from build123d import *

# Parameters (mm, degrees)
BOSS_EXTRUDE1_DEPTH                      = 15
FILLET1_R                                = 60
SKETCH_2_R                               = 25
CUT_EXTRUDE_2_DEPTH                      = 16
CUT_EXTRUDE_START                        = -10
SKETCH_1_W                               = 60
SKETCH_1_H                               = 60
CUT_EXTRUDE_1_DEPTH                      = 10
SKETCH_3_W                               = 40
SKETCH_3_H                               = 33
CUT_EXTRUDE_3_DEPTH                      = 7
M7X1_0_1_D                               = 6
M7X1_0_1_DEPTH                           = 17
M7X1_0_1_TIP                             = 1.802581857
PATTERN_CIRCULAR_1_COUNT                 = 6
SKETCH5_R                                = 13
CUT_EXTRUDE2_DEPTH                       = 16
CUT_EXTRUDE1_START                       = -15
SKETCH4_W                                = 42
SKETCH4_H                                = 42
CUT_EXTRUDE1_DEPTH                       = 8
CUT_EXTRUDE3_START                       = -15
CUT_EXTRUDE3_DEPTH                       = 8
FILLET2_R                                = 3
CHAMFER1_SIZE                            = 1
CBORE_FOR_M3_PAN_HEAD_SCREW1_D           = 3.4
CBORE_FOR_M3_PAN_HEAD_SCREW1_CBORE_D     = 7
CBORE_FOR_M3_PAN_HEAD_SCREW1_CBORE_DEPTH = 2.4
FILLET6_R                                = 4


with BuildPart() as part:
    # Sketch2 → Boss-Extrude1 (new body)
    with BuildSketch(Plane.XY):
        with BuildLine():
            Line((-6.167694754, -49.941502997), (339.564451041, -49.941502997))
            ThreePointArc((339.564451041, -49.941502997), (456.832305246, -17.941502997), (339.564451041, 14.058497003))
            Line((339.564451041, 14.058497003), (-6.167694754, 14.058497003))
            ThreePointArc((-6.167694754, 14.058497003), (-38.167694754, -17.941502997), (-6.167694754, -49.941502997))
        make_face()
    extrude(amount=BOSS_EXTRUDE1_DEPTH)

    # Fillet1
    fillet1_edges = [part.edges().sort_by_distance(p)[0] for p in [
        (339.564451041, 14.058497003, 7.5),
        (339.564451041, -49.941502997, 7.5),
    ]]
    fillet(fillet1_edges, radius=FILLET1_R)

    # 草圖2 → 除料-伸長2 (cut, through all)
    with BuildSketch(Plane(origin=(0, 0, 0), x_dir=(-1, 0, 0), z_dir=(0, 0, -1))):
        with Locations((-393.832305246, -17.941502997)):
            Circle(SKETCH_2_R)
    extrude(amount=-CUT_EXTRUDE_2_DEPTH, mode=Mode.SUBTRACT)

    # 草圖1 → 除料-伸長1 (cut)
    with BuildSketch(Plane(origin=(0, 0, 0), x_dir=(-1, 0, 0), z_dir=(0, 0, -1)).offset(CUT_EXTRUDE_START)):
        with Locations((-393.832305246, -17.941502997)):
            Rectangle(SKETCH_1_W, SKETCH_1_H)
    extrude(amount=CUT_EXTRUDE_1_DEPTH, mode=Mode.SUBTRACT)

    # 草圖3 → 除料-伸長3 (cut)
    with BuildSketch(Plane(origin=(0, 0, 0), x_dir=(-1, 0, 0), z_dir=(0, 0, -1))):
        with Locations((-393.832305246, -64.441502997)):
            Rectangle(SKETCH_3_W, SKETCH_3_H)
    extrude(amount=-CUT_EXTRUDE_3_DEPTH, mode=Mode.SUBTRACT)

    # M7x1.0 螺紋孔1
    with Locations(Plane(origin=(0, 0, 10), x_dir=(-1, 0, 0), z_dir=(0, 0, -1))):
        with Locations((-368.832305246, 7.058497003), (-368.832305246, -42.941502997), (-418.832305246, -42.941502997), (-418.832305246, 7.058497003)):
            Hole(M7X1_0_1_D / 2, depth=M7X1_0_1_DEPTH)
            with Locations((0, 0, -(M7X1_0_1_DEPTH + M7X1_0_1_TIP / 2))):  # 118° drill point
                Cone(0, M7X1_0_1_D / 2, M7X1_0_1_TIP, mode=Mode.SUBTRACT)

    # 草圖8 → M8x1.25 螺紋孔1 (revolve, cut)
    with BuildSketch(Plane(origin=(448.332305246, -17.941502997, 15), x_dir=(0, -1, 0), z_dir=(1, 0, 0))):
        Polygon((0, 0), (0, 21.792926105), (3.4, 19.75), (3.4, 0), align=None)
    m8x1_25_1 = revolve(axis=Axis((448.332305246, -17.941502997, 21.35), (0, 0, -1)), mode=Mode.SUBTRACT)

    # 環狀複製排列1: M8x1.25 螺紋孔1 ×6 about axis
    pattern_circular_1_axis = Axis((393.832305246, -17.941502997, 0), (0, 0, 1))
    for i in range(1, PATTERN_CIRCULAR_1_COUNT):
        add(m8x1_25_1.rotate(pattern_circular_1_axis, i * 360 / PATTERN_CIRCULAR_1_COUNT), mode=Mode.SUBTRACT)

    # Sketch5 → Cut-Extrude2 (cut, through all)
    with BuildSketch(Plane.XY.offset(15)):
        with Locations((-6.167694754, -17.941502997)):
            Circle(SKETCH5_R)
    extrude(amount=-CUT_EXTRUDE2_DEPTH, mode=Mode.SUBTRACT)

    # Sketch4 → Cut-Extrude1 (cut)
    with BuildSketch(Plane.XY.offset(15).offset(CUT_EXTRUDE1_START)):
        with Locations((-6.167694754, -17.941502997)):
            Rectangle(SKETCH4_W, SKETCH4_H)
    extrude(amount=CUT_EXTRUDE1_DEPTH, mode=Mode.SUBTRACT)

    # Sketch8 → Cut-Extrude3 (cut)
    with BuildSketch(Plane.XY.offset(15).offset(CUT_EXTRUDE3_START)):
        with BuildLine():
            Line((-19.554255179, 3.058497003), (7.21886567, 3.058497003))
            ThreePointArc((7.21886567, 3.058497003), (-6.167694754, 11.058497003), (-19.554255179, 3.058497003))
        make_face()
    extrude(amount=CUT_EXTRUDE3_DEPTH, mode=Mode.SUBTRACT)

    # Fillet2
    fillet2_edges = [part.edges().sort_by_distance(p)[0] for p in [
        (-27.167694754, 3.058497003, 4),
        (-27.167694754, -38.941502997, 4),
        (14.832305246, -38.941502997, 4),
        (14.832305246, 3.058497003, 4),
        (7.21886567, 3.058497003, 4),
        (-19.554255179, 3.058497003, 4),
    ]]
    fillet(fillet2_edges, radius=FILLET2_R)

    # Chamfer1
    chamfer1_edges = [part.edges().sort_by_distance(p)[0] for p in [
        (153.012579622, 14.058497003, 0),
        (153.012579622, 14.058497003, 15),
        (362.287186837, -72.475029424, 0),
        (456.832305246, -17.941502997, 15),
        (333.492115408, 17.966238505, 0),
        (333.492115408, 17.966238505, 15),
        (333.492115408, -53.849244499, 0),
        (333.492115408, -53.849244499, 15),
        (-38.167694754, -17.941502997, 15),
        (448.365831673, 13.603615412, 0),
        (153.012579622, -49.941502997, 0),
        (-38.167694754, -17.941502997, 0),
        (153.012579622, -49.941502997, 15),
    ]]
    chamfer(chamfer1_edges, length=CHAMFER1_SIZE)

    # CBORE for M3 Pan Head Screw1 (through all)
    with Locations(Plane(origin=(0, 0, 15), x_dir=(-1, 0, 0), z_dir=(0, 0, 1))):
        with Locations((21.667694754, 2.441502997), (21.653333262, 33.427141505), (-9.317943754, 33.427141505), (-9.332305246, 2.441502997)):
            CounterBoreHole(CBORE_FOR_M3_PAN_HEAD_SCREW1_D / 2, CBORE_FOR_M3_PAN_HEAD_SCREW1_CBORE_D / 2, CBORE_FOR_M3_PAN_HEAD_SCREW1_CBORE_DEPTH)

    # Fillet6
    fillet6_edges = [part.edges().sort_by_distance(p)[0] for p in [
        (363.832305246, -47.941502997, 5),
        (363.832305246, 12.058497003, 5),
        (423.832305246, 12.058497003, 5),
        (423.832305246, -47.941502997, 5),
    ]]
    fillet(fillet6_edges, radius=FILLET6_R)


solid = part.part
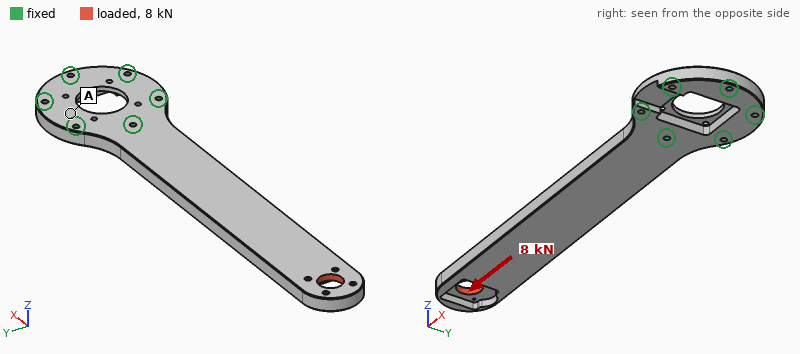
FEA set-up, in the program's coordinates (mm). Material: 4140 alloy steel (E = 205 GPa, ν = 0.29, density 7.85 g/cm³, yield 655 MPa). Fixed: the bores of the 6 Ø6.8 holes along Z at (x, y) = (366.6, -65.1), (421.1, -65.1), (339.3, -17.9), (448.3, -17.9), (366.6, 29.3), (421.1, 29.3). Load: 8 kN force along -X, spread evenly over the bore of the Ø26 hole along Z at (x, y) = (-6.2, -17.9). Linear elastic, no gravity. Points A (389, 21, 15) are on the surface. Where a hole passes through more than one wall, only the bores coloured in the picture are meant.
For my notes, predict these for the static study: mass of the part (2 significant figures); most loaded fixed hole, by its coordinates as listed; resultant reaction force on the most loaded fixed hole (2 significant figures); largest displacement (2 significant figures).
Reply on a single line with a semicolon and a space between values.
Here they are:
3.6 kg; (339.3, -17.9); 5.4 kN; 0.62 mm
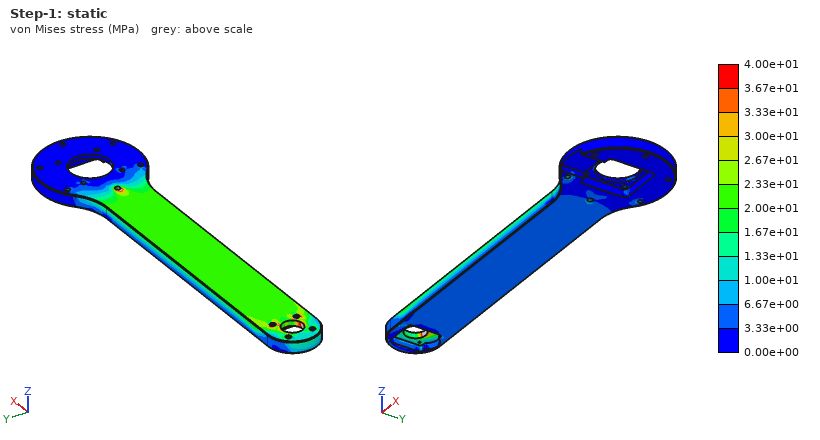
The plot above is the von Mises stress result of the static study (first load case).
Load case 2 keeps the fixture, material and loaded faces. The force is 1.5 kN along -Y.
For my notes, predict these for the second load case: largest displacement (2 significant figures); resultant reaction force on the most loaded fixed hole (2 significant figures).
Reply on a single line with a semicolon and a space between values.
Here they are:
0.41 mm; 5.6 kN
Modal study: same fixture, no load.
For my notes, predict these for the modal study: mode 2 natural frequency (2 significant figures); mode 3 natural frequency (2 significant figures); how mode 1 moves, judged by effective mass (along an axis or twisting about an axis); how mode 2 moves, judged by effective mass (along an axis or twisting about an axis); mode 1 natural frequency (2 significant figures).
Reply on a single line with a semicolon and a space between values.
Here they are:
380 Hz; 580 Hz; along Z; along Y; 98 Hz
